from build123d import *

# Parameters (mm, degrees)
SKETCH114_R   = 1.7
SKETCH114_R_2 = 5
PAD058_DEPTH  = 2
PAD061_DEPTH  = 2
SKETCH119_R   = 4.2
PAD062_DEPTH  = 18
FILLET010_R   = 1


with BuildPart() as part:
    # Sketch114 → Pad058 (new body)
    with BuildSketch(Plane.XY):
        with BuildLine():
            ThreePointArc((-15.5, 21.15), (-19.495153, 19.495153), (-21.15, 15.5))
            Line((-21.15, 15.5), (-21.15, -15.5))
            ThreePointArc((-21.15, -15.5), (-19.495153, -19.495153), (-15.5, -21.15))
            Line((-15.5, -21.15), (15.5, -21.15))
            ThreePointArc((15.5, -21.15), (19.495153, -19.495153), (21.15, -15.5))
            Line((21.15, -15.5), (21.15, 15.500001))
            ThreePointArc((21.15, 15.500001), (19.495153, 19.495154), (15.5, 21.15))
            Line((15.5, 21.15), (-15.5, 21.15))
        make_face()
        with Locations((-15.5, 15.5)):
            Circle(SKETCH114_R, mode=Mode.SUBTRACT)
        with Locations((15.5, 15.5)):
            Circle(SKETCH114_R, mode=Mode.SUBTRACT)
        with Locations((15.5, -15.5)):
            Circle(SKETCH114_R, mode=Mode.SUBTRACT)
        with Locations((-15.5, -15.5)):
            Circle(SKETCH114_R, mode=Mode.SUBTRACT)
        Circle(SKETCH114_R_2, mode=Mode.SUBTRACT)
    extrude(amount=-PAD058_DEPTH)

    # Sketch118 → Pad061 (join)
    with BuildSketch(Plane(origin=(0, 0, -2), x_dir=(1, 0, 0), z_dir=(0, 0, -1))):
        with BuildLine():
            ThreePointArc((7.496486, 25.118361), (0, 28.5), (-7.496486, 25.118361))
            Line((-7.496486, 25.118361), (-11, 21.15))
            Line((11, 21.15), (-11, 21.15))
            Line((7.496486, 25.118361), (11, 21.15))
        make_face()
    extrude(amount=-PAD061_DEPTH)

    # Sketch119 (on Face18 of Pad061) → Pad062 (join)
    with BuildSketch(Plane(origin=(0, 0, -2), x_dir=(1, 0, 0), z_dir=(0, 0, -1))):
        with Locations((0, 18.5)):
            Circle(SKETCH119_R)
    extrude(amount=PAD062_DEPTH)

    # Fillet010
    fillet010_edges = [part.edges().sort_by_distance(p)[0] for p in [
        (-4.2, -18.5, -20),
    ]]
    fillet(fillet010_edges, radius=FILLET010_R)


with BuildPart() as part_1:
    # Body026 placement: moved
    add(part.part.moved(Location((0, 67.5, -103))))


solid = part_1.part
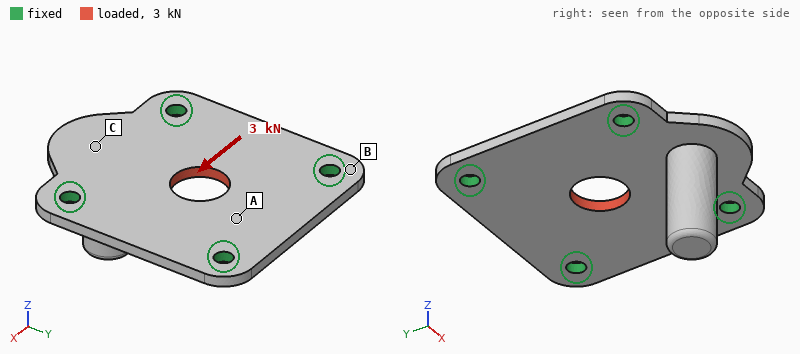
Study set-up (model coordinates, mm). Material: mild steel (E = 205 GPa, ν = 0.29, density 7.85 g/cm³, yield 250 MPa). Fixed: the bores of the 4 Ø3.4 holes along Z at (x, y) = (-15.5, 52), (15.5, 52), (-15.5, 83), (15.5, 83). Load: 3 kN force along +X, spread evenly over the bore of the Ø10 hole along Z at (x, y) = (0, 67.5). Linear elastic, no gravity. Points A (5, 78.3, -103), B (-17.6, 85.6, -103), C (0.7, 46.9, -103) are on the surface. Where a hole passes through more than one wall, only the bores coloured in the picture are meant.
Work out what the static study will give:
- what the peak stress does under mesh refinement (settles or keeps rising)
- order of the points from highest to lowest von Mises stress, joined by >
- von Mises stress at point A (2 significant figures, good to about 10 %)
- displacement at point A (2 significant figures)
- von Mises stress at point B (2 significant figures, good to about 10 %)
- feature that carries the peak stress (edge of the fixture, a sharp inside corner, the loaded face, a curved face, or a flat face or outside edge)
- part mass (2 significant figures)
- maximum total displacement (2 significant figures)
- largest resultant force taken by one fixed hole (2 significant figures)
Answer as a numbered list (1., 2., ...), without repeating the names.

1. keeps rising
2. A > B > C
3. 32 MPa
4. 1.9 µm
5. 16 MPa
6. edge of the fixture
7. 35 g
8. 4.6 µm
9. 820 N
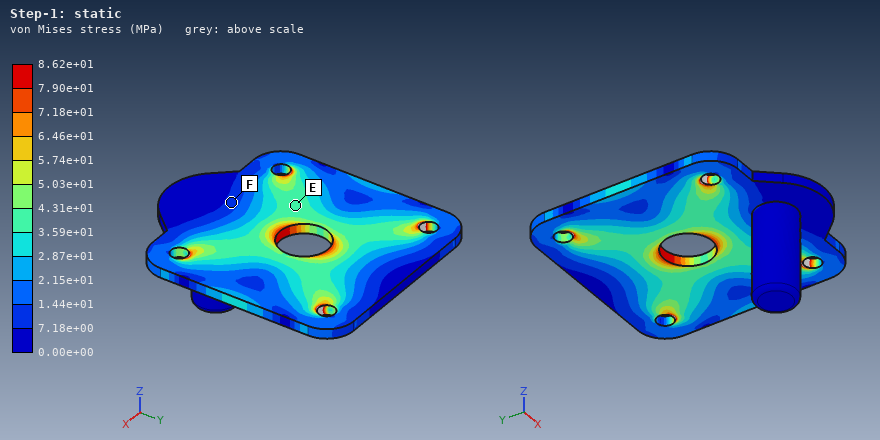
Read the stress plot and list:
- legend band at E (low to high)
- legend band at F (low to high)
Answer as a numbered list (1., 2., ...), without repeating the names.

1. 3.59e+01 to 4.31e+01 MPa
2. 7.18e+00 to 1.44e+01 MPa
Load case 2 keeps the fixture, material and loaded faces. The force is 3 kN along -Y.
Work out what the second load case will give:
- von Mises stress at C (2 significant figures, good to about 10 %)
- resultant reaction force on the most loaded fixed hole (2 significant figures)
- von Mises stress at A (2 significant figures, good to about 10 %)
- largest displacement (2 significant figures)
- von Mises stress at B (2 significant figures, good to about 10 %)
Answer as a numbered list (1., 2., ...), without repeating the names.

1. 14 MPa
2. 810 N
3. 32 MPa
4. 4.6 µm
5. 16 MPa
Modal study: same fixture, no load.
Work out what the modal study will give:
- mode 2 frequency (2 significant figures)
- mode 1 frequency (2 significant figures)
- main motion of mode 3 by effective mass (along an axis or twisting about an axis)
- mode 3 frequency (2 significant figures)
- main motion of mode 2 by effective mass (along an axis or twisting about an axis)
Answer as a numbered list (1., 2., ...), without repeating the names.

1. 6400 Hz
2. 3600 Hz
3. along Z
4. 6900 Hz
5. along X
